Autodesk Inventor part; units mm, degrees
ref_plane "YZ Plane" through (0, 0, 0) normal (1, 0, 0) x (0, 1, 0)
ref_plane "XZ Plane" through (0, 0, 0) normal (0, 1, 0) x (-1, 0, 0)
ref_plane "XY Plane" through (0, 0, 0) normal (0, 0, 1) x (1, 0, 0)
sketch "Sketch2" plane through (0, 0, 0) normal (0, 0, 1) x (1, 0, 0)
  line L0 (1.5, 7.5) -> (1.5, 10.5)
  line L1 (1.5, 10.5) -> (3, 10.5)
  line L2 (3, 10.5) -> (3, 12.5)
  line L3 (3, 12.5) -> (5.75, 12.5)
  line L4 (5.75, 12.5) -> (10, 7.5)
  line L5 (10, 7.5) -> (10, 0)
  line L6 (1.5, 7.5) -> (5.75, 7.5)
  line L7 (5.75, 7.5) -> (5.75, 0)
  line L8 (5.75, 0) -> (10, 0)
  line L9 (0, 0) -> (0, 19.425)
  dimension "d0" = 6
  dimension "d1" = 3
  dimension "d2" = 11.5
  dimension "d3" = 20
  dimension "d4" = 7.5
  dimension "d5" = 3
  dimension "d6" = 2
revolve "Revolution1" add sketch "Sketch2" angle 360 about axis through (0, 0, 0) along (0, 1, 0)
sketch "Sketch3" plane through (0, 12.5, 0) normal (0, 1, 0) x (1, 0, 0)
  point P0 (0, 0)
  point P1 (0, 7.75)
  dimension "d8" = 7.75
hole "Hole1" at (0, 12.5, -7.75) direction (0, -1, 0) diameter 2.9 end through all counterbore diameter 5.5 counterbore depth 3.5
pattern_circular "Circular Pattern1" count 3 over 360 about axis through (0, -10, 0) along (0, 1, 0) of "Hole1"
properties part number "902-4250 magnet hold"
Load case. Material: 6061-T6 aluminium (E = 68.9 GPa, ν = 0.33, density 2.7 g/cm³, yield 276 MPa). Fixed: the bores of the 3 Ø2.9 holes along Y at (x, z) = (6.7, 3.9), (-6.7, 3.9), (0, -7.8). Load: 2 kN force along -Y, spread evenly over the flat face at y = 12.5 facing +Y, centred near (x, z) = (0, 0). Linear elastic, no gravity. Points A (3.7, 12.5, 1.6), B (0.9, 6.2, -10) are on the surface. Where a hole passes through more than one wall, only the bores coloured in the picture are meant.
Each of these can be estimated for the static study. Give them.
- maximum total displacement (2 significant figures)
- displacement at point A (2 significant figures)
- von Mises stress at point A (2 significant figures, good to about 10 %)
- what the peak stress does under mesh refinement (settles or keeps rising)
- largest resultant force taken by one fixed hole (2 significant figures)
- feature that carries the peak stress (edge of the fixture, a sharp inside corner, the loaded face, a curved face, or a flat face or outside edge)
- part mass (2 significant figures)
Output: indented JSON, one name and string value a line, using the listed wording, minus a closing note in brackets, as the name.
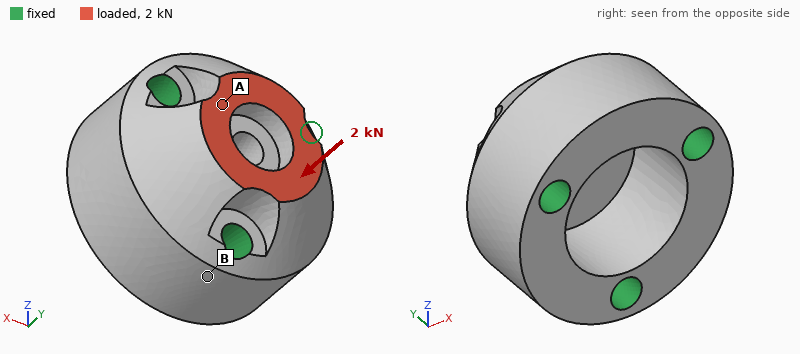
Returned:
{
  "maximum total displacement": "5.1 µm",
  "displacement at point A": "4.5 µm",
  "von Mises stress at point A": "29 MPa",
  "what the peak stress does under mesh refinement": "keeps rising",
  "largest resultant force taken by one fixed hole": "710 N",
  "feature that carries the peak stress": "edge of the fixture",
  "part mass": "6.0 g"
}
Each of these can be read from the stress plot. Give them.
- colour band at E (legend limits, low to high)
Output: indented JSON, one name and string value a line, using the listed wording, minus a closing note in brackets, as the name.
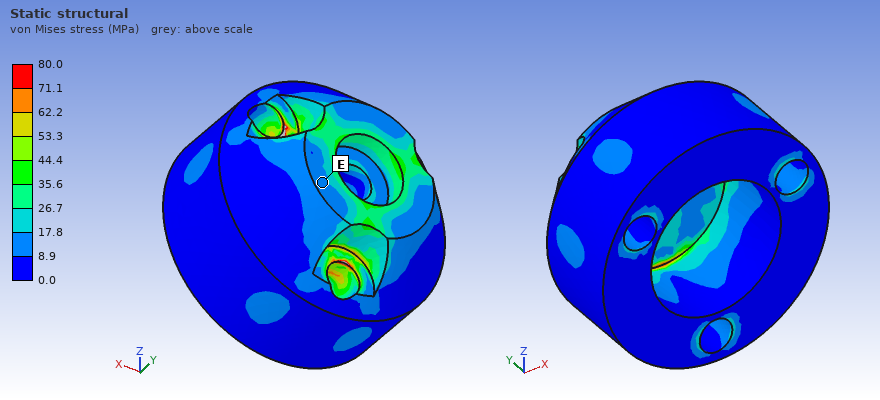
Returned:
{
  "colour band at E": "8.9 to 17.8 MPa"
}
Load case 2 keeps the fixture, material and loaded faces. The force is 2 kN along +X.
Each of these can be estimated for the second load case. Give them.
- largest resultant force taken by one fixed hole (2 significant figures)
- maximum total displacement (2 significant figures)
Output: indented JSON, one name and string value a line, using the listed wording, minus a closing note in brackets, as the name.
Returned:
{
  "largest resultant force taken by one fixed hole": "930 N",
  "maximum total displacement": "9.3 µm"
}
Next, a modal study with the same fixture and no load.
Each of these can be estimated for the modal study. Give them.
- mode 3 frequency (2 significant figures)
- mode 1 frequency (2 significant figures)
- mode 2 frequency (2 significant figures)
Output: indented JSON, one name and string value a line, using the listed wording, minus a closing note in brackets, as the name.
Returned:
{
  "mode 3 frequency": "82 kHz",
  "mode 1 frequency": "81 kHz",
  "mode 2 frequency": "81 kHz"
}
